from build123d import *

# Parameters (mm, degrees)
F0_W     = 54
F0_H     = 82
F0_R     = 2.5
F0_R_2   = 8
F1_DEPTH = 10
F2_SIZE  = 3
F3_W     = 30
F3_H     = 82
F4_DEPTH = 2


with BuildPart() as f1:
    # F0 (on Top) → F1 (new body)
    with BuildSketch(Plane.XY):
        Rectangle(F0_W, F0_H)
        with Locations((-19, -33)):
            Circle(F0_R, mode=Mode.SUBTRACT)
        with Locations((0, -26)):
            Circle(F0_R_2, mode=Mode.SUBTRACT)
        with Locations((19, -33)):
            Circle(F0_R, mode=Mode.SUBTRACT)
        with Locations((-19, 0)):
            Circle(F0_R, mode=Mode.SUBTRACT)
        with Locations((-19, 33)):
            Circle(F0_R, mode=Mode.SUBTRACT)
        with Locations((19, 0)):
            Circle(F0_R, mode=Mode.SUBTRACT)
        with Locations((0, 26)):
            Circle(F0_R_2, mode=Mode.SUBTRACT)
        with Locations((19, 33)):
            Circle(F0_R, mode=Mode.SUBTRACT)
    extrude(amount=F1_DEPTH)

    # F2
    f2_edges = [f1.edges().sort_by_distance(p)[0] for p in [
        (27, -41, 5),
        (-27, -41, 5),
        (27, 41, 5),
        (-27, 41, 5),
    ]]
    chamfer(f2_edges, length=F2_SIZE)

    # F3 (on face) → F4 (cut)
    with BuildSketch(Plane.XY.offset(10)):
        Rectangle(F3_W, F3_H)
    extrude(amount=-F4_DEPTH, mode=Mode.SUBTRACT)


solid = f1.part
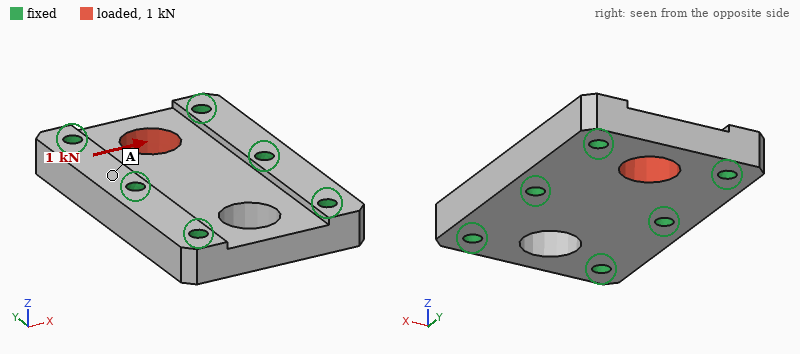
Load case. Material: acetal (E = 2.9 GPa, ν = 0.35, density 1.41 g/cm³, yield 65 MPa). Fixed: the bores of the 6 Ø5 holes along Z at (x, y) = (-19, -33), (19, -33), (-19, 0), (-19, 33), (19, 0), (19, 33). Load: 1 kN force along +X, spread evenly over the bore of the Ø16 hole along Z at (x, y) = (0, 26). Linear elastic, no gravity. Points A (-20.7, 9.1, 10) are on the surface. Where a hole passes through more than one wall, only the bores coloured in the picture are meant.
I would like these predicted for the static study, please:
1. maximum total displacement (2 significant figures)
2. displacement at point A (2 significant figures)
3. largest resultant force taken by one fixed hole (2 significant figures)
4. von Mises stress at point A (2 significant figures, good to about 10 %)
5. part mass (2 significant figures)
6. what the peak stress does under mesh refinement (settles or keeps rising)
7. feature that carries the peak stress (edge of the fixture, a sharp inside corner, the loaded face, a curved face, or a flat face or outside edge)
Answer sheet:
18 µm
6.1 µm
360 N
0.85 MPa
49 g
keeps rising
edge of the fixture
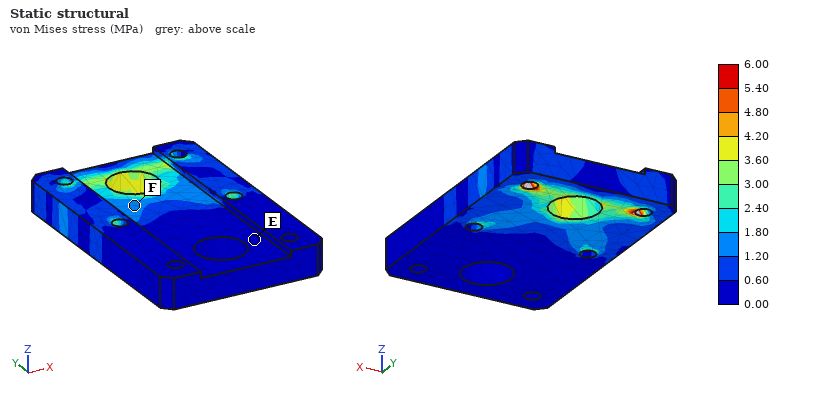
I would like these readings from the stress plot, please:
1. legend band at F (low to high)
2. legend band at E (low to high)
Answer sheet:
1.20 to 1.80 MPa
0.00 to 0.60 MPa
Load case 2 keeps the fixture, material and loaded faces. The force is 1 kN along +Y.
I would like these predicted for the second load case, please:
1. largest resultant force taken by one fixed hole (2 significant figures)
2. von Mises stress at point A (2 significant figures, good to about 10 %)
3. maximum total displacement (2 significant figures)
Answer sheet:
280 N
0.83 MPa
47 µm
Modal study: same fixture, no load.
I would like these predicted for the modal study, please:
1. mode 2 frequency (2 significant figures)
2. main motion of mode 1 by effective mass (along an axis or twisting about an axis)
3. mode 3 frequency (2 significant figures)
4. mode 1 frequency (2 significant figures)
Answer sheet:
6900 Hz
along Z
8200 Hz
6100 Hz
